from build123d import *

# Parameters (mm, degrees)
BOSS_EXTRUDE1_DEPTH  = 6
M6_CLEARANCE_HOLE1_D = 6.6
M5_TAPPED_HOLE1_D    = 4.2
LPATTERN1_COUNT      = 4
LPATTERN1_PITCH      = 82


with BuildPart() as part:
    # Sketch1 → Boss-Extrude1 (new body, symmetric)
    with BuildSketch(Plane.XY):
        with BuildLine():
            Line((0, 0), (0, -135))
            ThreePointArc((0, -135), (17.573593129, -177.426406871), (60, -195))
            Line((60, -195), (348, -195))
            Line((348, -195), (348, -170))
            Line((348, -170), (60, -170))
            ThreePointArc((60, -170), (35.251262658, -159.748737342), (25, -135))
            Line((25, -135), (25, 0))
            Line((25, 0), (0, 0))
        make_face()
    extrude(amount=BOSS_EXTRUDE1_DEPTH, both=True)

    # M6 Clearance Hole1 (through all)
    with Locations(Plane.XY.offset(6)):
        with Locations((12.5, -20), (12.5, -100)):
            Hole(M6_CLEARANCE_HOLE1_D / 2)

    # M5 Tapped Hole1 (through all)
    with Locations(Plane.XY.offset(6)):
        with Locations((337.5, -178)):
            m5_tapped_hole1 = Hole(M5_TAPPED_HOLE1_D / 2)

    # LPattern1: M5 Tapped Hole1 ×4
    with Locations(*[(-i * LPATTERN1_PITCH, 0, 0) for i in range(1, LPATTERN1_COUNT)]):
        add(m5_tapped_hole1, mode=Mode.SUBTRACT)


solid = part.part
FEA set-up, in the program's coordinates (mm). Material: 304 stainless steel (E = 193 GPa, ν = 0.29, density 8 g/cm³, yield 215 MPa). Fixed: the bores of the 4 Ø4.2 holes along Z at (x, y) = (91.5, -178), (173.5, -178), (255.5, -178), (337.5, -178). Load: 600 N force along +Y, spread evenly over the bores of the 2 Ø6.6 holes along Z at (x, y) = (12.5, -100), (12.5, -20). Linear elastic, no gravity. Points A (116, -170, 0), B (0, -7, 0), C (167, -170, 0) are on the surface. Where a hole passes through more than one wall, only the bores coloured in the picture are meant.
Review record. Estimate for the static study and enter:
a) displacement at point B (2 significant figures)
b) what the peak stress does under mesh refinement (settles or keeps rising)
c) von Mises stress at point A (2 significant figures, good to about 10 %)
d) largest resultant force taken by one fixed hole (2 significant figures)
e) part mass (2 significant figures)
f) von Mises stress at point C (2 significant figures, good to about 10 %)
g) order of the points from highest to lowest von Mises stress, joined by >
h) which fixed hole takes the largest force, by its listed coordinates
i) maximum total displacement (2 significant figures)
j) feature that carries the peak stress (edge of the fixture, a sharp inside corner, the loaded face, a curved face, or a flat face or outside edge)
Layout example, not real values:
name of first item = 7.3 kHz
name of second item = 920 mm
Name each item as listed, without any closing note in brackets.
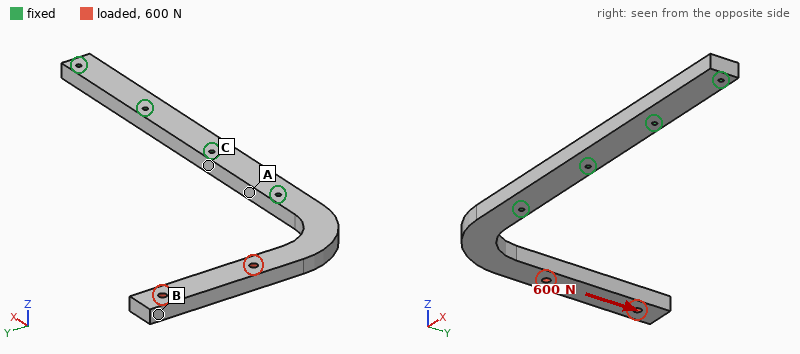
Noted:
displacement at point B = 0.17 mm
what the peak stress does under mesh refinement = keeps rising
von Mises stress at point A = 12 MPa
largest resultant force taken by one fixed hole = 1.4 kN
part mass = 1.2 kg
von Mises stress at point C = 6.4 MPa
order of the points from highest to lowest von Mises stress, joined by > = A > C > B
which fixed hole takes the largest force, by its listed coordinates = (91.5, -178)
maximum total displacement = 0.18 mm
feature that carries the peak stress = edge of the fixture
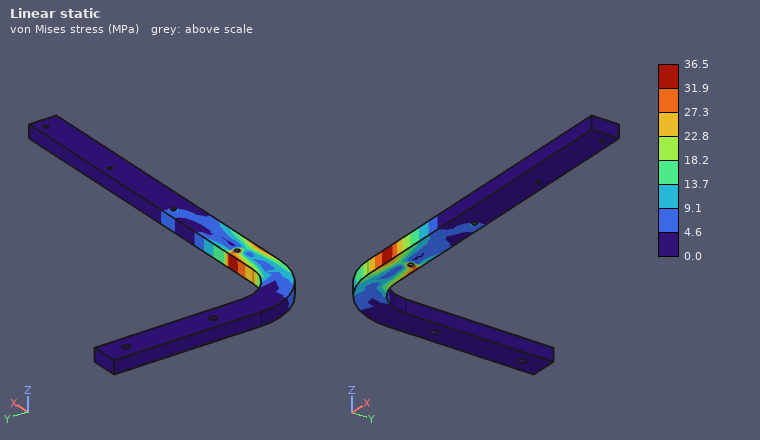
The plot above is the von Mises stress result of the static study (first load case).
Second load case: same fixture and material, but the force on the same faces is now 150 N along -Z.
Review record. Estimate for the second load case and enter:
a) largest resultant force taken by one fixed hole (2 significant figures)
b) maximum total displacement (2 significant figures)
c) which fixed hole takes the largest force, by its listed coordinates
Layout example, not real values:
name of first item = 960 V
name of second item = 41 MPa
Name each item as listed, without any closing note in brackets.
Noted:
largest resultant force taken by one fixed hole = 160 N
maximum total displacement = 0.54 mm
which fixed hole takes the largest force, by its listed coordinates = (91.5, -178)
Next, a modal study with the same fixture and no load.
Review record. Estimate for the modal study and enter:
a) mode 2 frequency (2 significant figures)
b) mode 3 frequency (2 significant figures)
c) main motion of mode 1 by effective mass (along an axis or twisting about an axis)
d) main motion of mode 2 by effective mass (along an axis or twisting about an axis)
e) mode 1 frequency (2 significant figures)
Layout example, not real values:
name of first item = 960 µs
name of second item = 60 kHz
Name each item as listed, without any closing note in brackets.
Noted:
mode 2 frequency = 350 Hz
mode 3 frequency = 790 Hz
main motion of mode 1 by effective mass = along Z
main motion of mode 2 by effective mass = along X
mode 1 frequency = 190 Hz
